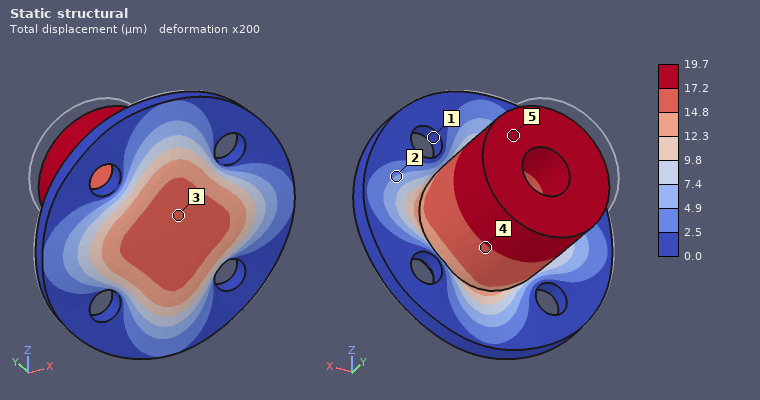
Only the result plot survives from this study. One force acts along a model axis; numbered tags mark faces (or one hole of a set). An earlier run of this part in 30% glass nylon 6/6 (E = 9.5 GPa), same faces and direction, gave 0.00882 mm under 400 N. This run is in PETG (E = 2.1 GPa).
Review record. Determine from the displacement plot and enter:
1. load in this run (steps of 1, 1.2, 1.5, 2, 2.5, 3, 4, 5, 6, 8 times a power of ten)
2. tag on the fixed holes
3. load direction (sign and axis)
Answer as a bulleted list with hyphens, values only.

- 200 N
- 1
- -Y
